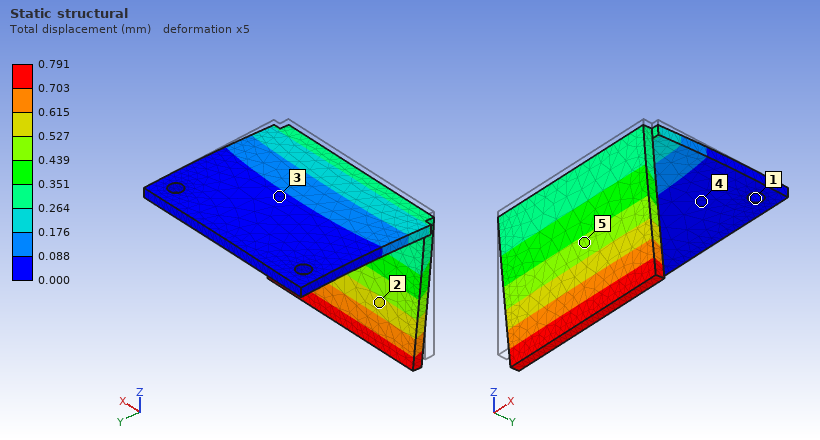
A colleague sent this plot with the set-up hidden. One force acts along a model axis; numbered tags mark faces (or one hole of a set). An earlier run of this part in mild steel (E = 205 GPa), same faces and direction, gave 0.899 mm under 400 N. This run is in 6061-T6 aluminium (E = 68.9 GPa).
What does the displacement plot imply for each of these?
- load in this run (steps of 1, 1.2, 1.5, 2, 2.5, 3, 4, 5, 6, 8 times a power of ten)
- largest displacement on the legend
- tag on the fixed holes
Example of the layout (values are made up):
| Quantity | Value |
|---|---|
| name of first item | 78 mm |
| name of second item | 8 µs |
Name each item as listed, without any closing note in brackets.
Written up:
| Quantity | Value |
|---|---|
| load in this run | 120 N |
| largest displacement on the legend | 0.791 mm |
| tag on the fixed holes | 1 |
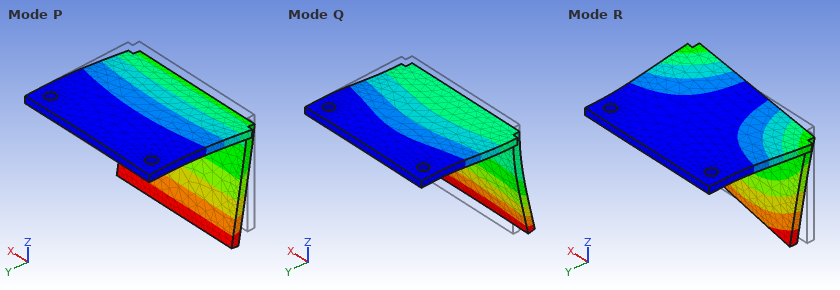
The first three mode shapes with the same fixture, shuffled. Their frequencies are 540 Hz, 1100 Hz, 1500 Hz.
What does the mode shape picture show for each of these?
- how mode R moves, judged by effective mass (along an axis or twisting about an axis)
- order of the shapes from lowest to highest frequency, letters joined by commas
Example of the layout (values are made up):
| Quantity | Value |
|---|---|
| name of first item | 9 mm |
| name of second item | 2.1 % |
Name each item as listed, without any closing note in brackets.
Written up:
| Quantity | Value |
|---|---|
| how mode R moves, judged by effective mass | along X |
| order of the shapes from lowest to highest frequency, letters joined by commas | P, R, Q |
